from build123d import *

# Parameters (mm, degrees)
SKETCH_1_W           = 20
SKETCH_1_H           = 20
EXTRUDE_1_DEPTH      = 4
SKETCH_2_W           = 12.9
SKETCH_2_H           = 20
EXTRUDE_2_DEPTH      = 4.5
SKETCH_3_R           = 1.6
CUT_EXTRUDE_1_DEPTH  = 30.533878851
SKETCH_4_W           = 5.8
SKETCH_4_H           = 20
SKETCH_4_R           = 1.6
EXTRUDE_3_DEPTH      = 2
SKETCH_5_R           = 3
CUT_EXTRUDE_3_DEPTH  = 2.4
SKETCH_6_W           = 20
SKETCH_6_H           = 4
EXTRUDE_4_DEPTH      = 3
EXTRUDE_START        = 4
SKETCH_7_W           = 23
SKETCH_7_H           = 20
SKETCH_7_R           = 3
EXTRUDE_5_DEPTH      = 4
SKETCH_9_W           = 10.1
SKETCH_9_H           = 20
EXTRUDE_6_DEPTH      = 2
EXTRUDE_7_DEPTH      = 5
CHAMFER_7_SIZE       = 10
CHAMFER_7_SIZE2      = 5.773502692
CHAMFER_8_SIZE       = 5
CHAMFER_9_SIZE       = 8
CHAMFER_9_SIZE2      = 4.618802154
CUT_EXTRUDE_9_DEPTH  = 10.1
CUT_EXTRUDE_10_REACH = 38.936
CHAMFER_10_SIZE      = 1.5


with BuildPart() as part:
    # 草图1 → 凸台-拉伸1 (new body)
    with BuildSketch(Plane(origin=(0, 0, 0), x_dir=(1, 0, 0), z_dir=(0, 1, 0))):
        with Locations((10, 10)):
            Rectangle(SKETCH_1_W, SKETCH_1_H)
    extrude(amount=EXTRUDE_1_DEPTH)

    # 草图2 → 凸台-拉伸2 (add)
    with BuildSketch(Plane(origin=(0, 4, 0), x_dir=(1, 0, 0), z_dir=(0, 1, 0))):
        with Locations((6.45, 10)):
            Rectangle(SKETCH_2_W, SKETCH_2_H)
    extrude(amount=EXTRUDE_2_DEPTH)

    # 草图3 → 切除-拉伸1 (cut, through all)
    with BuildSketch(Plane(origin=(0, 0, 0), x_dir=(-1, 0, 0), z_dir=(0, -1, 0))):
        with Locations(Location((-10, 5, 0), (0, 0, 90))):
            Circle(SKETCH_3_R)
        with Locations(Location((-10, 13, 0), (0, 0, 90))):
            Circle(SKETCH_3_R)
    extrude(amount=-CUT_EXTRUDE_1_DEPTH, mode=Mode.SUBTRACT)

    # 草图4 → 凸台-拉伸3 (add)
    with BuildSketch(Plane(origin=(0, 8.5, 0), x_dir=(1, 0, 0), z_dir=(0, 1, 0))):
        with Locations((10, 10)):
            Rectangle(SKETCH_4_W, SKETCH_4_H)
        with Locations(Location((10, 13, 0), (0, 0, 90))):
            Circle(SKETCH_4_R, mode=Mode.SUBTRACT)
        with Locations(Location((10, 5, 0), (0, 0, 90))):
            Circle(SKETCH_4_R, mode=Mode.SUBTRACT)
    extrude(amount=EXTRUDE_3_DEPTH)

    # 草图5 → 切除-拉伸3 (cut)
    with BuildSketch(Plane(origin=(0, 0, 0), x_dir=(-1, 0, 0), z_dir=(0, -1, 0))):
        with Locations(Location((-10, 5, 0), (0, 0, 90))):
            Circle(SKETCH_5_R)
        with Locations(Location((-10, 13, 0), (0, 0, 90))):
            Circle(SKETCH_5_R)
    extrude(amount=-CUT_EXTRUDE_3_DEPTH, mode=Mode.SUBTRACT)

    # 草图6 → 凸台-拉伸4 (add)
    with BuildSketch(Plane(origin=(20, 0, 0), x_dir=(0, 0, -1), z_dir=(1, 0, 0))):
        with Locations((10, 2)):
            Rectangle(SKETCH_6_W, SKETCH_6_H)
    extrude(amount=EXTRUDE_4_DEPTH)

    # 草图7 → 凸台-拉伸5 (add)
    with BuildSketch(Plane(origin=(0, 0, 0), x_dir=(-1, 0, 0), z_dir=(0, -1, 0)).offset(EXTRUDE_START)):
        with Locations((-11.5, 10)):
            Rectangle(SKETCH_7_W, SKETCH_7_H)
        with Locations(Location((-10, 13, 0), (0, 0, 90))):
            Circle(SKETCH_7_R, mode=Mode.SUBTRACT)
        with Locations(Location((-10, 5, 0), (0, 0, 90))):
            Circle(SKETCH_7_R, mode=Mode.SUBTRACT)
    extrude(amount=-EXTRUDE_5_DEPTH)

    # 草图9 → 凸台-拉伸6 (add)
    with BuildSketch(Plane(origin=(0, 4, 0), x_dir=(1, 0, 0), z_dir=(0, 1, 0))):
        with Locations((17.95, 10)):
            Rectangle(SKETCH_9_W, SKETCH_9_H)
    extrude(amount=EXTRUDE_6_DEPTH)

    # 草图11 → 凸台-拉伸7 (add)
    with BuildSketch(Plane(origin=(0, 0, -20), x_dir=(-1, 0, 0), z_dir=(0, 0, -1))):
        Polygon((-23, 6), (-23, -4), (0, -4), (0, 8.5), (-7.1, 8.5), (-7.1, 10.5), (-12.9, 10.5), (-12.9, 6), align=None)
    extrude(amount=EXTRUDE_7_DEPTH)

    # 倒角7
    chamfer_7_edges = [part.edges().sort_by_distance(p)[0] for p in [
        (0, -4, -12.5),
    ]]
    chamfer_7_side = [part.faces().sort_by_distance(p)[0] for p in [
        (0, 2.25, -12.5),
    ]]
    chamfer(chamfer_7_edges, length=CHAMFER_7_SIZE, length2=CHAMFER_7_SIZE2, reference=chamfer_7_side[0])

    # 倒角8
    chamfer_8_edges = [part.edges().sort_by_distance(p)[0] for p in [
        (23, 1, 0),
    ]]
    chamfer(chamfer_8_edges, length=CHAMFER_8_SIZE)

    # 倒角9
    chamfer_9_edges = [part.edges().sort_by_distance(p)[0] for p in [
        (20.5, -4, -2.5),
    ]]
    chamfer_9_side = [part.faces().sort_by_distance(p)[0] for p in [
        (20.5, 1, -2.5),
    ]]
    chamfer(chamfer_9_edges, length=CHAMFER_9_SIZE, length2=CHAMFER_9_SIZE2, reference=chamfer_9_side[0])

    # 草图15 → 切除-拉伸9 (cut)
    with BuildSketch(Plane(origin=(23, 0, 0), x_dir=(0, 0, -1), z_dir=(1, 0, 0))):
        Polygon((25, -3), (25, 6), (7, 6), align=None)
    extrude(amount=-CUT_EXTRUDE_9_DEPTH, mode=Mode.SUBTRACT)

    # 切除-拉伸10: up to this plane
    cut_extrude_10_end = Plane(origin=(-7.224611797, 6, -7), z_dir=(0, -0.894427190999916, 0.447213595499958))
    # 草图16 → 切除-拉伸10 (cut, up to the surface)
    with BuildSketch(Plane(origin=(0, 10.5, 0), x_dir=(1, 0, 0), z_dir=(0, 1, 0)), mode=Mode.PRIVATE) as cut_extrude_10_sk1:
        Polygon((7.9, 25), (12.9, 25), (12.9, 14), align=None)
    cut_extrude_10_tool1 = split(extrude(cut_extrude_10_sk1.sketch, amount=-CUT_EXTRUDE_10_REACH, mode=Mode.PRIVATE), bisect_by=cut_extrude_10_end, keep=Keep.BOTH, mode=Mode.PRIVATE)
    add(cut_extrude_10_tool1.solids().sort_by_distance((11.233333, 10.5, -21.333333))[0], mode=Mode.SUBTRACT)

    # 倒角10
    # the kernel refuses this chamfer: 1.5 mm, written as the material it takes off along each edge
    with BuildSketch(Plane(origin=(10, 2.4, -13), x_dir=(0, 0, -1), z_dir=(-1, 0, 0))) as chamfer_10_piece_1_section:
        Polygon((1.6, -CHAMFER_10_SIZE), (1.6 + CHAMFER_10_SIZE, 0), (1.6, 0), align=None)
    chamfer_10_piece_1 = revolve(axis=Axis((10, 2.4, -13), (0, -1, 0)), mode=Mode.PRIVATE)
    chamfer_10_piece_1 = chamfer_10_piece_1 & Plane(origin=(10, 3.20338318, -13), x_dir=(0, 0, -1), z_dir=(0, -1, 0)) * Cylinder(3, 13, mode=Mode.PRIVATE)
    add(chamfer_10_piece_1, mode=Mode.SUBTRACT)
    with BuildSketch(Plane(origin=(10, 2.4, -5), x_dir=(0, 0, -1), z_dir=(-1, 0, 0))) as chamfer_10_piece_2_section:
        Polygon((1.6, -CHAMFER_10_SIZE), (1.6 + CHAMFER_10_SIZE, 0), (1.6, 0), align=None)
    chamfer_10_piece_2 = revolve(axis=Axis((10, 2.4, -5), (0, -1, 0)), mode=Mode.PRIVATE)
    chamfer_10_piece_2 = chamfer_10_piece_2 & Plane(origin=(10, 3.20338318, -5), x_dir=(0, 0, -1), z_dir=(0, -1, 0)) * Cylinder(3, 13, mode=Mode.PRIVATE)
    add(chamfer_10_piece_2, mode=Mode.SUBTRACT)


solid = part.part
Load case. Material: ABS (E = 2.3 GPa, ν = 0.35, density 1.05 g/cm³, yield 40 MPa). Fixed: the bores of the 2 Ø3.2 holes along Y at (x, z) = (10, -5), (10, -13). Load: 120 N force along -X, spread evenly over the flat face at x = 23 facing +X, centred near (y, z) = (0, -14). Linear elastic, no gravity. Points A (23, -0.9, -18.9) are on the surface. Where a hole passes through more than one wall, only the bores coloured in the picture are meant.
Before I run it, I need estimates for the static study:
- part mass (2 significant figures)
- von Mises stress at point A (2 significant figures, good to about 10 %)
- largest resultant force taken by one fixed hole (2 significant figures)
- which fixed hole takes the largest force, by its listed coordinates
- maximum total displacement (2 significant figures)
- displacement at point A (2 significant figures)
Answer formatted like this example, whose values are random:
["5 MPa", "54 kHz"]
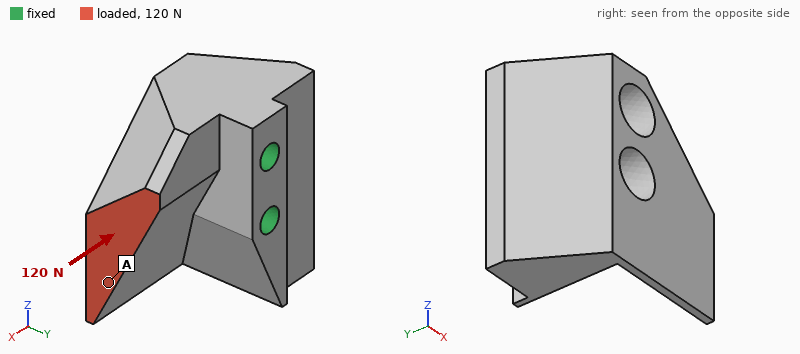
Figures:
["4.4 g", "1.2 MPa", "110 N", "(10, -13)", "82 µm", "67 µm"]
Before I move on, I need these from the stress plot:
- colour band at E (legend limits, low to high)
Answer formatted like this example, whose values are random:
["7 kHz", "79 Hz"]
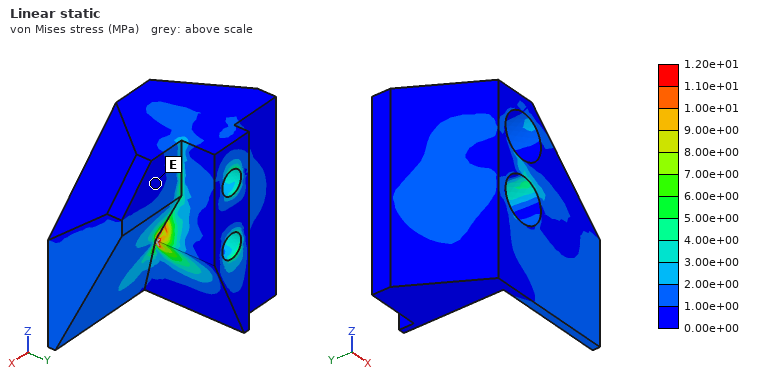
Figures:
["0.00e+00 to 1.00e+00 MPa"]
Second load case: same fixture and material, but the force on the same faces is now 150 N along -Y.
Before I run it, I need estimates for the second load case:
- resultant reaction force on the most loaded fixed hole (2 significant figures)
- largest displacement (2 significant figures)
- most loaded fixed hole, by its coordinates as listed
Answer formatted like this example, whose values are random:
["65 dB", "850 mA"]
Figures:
["140 N", "0.41 mm", "(10, -13)"]
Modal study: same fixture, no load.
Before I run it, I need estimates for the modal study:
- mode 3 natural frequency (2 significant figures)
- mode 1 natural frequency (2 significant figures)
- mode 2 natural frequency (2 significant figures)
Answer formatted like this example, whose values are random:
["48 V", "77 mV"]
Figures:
["7800 Hz", "4400 Hz", "5900 Hz"]
